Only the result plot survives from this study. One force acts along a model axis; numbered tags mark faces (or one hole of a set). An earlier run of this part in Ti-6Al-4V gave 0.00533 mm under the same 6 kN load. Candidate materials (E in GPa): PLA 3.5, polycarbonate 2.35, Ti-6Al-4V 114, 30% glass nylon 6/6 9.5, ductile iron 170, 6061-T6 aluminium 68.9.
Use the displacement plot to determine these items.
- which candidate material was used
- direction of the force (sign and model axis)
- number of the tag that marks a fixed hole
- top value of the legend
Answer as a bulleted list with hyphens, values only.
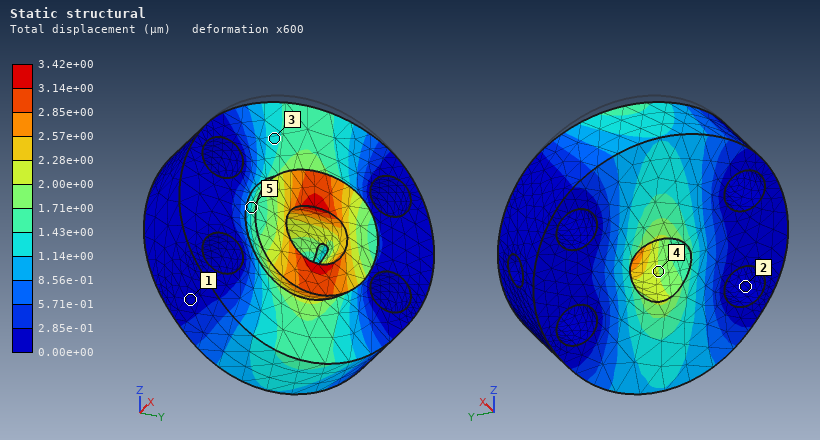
- ductile iron
- -Z
- 2
- 3.42e+00 µm
